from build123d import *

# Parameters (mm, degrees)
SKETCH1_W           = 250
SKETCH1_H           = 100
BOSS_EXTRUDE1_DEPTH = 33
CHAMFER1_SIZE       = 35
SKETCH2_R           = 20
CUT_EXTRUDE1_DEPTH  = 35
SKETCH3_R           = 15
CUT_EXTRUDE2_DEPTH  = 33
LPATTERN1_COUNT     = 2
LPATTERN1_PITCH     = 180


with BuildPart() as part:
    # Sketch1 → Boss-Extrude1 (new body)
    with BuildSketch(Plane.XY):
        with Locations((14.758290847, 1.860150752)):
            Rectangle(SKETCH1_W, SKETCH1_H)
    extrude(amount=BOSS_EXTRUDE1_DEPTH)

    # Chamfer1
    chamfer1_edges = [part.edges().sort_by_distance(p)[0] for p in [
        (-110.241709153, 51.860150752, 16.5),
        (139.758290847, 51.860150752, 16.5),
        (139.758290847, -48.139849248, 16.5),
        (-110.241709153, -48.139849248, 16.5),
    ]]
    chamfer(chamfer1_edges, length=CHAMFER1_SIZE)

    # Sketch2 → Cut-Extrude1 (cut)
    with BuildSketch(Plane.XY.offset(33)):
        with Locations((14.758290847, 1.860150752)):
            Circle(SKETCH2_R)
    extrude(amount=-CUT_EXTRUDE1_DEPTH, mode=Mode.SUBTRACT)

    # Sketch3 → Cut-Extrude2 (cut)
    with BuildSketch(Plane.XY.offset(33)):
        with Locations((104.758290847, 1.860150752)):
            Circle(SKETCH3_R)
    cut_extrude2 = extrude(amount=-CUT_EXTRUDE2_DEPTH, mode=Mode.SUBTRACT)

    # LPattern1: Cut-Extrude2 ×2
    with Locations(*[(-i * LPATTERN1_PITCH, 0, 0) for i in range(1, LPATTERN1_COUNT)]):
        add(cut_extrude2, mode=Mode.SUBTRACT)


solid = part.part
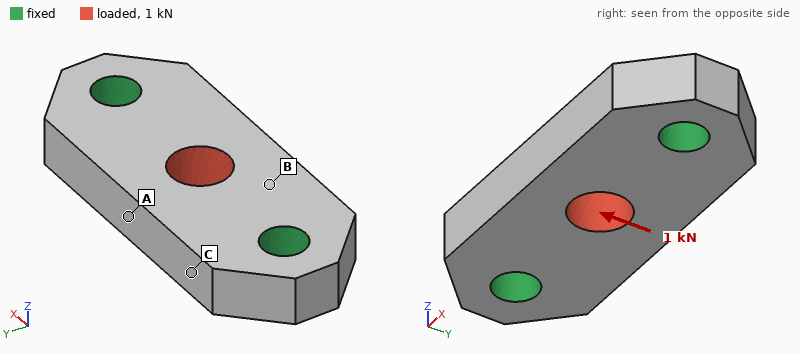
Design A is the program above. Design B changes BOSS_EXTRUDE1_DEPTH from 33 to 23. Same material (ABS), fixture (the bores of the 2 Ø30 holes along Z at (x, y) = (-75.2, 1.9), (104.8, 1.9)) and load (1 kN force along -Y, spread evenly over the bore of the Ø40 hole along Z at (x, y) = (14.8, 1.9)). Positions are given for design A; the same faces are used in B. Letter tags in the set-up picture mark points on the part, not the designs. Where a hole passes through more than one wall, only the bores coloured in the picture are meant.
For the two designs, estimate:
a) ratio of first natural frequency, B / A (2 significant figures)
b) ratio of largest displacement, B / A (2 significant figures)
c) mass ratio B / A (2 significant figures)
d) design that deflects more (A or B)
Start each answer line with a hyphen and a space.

- 0.79
- 1.4
- 0.70
- B
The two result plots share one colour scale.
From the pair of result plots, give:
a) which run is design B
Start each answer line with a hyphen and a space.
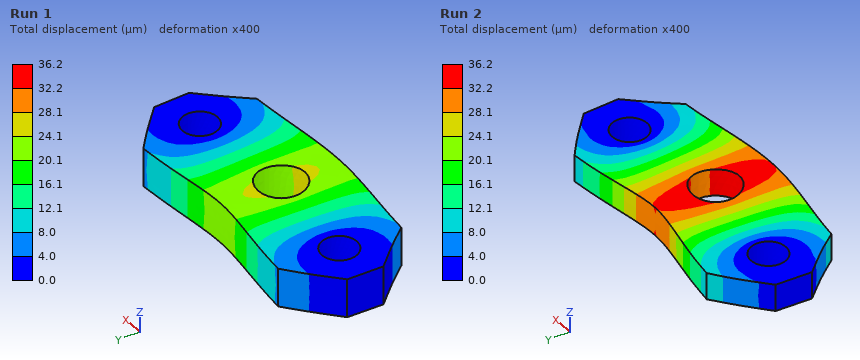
- Run 2
